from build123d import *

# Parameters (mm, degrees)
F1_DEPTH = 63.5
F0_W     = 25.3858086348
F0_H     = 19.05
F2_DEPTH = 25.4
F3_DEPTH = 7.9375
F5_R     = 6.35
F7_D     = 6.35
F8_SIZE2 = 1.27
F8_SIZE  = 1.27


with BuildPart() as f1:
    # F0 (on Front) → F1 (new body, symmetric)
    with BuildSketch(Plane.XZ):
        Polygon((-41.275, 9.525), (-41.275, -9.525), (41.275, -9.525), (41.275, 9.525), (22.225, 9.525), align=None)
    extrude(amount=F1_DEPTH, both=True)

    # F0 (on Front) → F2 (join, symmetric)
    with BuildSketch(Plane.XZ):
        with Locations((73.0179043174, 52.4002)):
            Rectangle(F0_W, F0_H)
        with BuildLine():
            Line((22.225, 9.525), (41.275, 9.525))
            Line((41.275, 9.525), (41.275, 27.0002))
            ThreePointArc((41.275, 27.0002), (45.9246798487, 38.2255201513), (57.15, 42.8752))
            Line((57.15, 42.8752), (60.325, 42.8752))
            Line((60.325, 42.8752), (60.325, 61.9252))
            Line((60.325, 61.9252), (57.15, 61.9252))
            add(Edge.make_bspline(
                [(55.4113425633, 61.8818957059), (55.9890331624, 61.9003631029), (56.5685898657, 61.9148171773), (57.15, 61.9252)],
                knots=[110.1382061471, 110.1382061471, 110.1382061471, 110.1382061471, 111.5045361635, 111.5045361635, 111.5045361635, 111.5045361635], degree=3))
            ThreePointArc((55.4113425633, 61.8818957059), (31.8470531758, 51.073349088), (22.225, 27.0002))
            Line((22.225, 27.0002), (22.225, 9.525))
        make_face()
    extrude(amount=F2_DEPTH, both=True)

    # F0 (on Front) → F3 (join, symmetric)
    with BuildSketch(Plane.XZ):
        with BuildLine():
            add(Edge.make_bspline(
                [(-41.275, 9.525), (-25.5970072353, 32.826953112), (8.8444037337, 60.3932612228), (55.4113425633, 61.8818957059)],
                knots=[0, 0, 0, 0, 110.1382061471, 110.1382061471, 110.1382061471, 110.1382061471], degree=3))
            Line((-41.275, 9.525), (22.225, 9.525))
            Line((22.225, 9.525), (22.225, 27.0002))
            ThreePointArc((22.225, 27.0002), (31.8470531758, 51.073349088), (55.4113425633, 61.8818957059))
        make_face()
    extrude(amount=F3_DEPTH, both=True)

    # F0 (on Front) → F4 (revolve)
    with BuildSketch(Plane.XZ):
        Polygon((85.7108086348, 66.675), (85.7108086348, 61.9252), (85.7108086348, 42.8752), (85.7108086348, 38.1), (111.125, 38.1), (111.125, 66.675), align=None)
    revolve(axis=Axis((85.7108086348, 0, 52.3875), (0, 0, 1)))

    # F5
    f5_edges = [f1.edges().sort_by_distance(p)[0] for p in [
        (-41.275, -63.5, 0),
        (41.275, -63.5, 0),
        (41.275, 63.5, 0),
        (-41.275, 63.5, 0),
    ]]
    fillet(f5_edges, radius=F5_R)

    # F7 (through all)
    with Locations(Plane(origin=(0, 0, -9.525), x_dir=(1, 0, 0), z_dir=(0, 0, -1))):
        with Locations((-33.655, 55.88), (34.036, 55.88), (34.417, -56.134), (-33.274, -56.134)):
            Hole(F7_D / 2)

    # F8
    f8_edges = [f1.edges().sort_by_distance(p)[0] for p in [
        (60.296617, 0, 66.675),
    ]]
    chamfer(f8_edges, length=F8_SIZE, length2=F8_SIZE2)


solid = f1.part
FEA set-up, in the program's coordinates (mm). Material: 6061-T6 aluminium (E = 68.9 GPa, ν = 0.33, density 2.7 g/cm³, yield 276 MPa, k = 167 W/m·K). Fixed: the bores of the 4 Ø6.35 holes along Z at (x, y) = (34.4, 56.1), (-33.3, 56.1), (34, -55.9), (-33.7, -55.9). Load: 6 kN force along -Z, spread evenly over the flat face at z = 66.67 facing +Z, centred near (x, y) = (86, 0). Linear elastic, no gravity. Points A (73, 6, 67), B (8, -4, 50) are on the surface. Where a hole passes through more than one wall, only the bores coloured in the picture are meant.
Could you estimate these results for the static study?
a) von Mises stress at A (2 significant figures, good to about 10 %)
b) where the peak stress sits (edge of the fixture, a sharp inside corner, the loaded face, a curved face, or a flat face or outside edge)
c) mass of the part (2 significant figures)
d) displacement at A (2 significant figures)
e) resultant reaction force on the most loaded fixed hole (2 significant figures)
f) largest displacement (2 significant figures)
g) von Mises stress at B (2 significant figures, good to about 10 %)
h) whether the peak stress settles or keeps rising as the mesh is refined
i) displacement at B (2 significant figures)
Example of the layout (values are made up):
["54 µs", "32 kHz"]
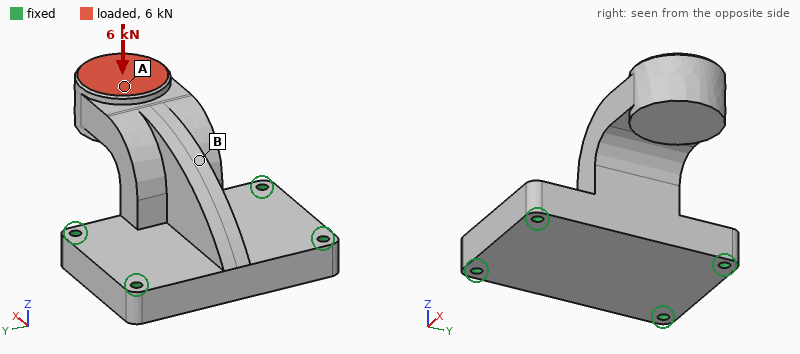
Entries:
["15 MPa", "edge of the fixture", "950 g", "0.29 mm", "5.5 kN", "0.49 mm", "39 MPa", "keeps rising", "0.074 mm"]
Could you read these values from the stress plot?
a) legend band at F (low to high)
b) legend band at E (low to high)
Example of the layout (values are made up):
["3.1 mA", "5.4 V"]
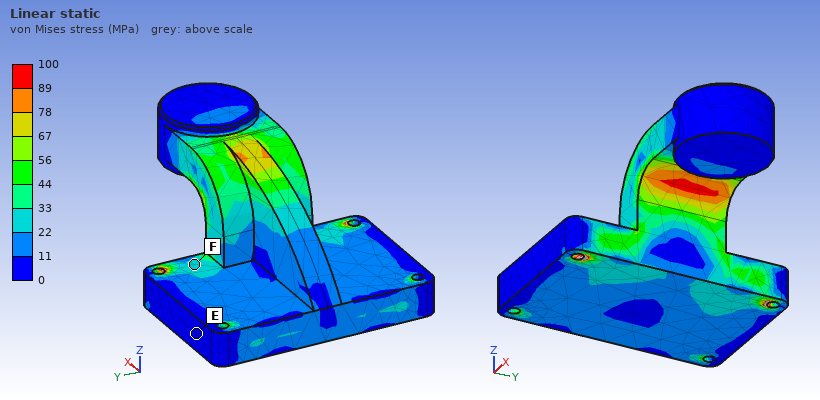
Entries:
["22 to 33 MPa", "0 to 11 MPa"]
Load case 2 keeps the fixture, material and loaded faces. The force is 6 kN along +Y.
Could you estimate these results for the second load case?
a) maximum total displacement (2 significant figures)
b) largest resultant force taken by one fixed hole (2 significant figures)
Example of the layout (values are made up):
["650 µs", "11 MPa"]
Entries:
["0.34 mm", "4.9 kN"]
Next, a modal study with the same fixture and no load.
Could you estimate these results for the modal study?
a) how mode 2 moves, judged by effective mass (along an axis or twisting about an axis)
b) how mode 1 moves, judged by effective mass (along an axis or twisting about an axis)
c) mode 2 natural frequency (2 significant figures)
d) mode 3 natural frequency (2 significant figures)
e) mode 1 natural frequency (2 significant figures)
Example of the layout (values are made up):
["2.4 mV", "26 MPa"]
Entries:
["along Y", "along Z", "1800 Hz", "3700 Hz", "1500 Hz"]
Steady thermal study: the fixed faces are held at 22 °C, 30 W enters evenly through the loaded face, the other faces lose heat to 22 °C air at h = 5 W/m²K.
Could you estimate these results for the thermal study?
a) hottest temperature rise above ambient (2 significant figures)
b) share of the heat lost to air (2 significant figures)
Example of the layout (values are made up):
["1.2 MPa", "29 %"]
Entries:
["18 K", "4.0 %"]
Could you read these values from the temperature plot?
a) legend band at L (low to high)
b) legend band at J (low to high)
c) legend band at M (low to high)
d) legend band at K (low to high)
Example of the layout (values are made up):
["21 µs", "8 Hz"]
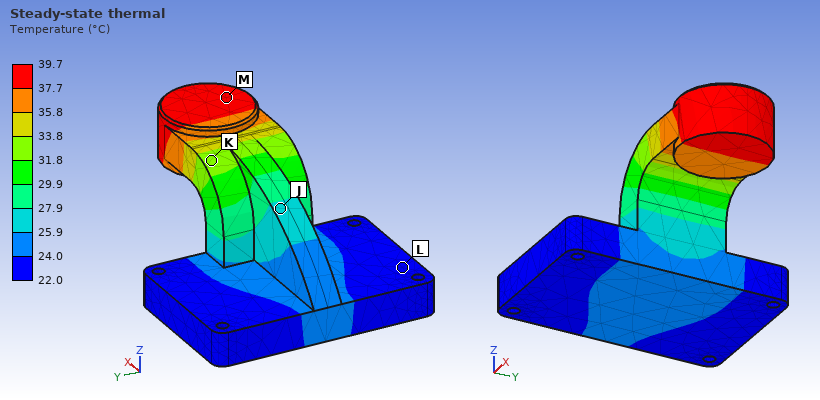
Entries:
["22.0 to 24.0 °C", "25.9 to 27.9 °C", "37.7 to 39.7 °C", "31.8 to 33.8 °C"]
